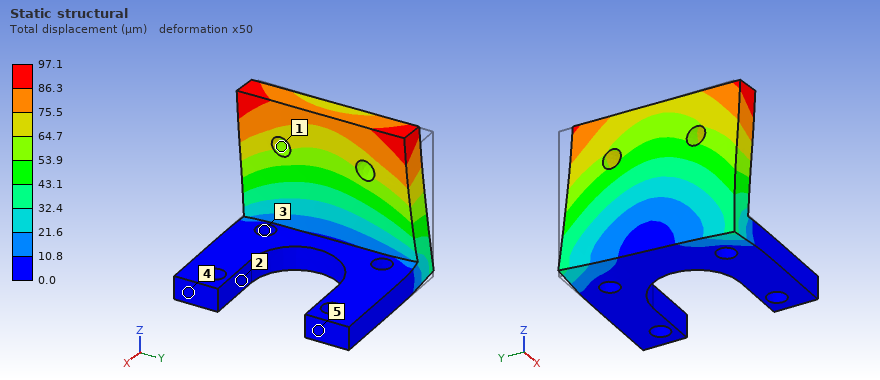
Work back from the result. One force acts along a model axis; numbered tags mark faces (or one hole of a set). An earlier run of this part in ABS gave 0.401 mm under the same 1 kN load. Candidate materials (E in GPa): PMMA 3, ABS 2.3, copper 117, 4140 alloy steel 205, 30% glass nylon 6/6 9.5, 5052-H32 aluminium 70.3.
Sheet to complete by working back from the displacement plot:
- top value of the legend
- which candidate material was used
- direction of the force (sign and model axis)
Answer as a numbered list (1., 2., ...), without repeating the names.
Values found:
1. 97.1 µm
2. 30% glass nylon 6/6
3. -Y
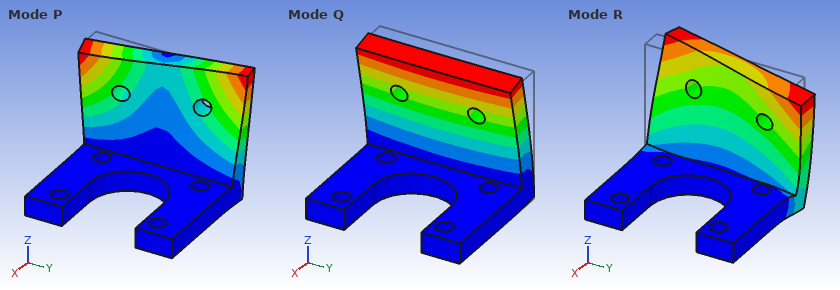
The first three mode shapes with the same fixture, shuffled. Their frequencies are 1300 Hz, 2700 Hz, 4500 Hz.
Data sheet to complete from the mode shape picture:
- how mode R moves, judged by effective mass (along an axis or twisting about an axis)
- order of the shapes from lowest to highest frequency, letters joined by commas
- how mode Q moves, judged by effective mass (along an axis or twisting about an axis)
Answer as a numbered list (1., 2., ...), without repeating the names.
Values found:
1. along Y
2. Q, P, R
3. along X
